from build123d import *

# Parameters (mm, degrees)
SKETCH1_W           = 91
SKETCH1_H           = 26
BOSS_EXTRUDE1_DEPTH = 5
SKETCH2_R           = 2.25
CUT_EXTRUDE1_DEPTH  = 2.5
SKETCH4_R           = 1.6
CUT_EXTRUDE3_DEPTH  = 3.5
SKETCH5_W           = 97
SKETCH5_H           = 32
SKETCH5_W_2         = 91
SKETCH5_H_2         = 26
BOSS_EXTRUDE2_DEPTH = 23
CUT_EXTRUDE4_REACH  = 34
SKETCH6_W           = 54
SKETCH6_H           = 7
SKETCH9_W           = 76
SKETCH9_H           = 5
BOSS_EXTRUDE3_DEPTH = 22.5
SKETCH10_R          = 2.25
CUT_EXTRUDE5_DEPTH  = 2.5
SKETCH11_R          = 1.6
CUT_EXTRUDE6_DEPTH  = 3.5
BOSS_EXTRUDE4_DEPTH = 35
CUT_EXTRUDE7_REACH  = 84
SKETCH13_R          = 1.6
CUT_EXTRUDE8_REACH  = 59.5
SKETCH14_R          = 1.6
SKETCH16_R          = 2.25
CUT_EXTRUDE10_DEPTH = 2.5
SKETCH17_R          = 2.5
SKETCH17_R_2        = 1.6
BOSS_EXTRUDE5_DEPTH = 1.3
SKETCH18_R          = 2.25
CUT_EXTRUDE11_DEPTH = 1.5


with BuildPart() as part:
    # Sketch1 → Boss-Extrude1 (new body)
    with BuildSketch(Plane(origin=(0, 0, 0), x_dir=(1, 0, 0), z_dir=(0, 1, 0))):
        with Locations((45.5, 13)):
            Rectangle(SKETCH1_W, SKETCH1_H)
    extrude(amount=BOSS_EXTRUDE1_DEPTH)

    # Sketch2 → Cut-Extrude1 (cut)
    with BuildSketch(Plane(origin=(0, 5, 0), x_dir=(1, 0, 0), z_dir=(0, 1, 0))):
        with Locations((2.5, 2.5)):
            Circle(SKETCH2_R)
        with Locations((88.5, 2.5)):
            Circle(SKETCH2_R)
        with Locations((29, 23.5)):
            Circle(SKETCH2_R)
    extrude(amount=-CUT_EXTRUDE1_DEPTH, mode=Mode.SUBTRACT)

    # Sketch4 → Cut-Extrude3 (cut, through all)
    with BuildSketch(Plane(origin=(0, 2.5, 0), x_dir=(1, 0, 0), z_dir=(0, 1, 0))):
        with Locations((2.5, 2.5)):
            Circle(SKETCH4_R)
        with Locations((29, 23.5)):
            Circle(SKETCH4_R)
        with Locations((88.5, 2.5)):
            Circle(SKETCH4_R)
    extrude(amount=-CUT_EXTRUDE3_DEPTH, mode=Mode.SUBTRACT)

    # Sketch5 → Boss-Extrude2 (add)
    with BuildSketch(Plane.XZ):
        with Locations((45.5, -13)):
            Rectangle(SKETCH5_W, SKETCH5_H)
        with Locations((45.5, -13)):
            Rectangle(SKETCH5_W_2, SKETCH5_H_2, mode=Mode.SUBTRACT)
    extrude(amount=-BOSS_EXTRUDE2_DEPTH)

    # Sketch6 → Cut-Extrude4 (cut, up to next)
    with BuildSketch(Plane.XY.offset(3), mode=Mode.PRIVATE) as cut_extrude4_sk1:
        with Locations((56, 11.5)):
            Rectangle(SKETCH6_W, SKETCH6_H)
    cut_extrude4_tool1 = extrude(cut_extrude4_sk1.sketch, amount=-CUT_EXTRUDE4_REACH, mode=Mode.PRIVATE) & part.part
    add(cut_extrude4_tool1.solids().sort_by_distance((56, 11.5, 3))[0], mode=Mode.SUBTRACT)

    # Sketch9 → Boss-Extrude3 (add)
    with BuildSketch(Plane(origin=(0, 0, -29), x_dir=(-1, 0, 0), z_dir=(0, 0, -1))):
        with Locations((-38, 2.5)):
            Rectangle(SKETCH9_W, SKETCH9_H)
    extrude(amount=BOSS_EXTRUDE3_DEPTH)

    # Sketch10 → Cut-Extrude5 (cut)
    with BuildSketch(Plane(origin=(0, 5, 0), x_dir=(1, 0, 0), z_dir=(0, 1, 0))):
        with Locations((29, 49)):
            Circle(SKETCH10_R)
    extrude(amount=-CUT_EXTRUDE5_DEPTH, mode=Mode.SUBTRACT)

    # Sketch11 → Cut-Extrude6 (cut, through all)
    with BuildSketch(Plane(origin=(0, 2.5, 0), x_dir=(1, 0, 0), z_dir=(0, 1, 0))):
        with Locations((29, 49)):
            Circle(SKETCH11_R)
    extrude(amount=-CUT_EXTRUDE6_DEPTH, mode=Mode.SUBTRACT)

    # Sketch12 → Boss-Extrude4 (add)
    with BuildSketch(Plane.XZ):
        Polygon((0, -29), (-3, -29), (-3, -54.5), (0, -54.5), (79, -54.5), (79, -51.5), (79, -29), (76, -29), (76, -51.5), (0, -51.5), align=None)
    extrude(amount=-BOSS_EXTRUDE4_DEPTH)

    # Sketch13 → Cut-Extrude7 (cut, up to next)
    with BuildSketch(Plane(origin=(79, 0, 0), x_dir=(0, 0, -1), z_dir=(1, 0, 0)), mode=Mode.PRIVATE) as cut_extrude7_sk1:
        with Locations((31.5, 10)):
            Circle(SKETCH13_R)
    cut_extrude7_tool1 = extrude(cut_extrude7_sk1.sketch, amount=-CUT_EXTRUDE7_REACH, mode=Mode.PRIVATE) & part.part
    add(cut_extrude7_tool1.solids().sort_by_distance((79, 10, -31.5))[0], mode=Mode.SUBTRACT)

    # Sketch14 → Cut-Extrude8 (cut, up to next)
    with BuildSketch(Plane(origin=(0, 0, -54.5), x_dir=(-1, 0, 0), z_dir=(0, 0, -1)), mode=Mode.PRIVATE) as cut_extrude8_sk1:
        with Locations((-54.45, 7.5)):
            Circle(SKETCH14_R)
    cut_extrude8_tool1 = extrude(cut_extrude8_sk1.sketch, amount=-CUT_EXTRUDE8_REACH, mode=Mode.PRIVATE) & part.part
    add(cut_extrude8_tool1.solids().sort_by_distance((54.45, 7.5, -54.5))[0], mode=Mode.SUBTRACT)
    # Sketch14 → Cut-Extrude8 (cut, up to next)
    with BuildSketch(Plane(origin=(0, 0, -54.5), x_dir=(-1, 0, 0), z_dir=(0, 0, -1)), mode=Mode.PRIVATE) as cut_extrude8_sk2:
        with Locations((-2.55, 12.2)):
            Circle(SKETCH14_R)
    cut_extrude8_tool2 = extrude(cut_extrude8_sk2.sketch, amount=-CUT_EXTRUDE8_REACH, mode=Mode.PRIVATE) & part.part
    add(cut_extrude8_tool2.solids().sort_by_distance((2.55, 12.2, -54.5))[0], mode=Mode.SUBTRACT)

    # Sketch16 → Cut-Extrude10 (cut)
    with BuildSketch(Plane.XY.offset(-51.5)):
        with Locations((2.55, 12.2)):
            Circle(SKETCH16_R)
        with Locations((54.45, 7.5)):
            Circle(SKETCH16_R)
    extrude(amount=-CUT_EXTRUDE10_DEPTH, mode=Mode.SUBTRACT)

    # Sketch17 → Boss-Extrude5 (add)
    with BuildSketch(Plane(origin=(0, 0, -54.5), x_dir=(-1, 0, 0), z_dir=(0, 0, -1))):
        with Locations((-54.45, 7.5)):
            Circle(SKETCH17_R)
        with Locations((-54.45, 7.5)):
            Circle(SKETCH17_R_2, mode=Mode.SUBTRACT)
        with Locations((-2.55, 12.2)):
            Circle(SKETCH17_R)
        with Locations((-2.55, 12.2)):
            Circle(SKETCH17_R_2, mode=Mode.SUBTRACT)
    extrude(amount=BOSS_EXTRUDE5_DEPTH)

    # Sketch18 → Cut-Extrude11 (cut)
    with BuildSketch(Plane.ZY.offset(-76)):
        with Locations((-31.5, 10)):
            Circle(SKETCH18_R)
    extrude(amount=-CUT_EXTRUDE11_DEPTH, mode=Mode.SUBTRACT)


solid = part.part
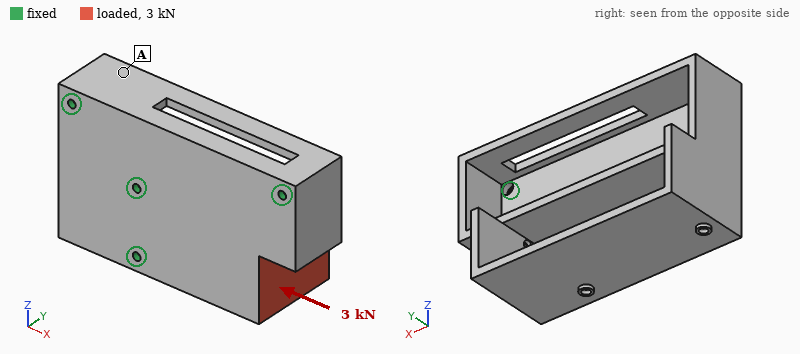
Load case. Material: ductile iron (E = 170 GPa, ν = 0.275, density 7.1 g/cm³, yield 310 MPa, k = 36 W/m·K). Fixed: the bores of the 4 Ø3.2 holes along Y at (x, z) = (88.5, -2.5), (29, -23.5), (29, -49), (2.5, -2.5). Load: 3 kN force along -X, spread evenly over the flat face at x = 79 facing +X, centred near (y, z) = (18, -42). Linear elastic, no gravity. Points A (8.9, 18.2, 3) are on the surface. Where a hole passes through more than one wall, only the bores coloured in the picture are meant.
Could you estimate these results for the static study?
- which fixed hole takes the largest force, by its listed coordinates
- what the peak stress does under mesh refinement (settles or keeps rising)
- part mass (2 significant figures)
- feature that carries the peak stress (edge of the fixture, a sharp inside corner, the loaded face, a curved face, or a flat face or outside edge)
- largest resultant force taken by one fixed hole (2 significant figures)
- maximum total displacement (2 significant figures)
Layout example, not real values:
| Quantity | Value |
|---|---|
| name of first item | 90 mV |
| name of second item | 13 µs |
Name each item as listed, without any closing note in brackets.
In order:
| Quantity | Value |
|---|---|
| which fixed hole takes the largest force, by its listed coordinates | (88.5, -2.5) |
| what the peak stress does under mesh refinement | keeps rising |
| part mass | 350 g |
| feature that carries the peak stress | edge of the fixture |
| largest resultant force taken by one fixed hole | 1.3 kN |
| maximum total displacement | 0.16 mm |
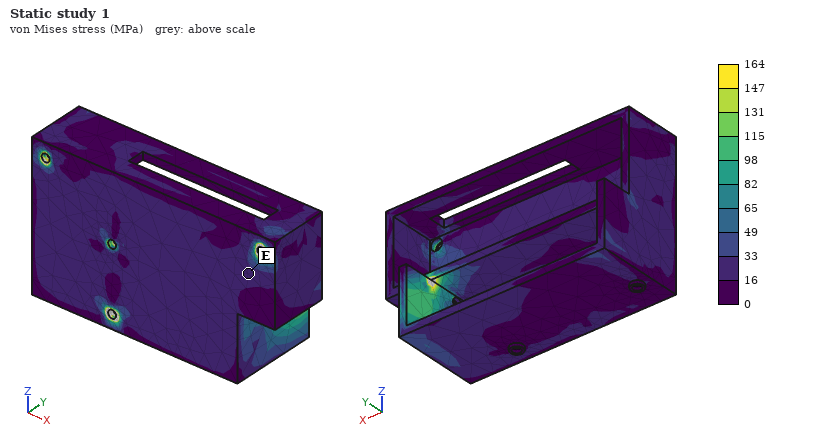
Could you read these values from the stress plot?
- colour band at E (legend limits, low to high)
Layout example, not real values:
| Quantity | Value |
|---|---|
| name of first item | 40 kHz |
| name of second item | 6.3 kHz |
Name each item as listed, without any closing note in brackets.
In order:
| Quantity | Value |
|---|---|
| colour band at E | 16 to 33 MPa |
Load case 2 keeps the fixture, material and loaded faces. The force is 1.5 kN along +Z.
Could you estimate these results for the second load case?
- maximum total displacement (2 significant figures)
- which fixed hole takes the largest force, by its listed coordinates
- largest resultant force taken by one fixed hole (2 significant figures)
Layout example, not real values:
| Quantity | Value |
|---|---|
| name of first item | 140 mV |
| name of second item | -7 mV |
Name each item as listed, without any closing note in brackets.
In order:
| Quantity | Value |
|---|---|
| maximum total displacement | 0.13 mm |
| which fixed hole takes the largest force, by its listed coordinates | (29, -49) |
| largest resultant force taken by one fixed hole | 1.1 kN |
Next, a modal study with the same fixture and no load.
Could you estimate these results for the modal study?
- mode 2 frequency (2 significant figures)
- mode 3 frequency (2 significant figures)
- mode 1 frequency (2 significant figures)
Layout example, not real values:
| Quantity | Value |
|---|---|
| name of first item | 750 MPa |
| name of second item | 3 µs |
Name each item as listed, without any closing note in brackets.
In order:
| Quantity | Value |
|---|---|
| mode 2 frequency | 2900 Hz |
| mode 3 frequency | 3400 Hz |
| mode 1 frequency | 1700 Hz |
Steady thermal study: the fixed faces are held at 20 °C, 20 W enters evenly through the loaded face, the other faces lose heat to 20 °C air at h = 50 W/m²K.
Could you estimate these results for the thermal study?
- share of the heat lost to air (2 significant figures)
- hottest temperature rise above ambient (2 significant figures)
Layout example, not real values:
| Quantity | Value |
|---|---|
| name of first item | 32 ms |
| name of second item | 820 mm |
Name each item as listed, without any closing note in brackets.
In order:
| Quantity | Value |
|---|---|
| share of the heat lost to air | 67 % |
| hottest temperature rise above ambient | 65 K |
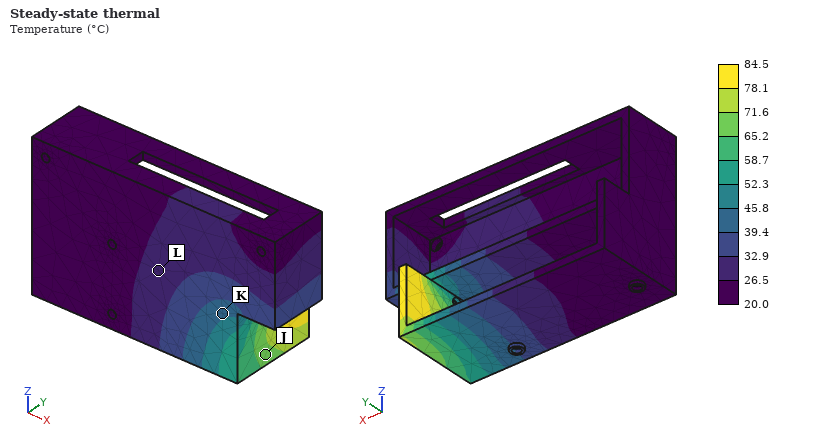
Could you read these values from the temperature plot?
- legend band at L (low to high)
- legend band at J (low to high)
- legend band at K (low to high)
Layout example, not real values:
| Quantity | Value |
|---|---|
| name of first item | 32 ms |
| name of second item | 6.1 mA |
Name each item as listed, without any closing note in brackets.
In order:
| Quantity | Value |
|---|---|
| legend band at L | 26.5 to 32.9 °C |
| legend band at J | 65.2 to 71.6 °C |
| legend band at K | 39.4 to 45.8 °C |
